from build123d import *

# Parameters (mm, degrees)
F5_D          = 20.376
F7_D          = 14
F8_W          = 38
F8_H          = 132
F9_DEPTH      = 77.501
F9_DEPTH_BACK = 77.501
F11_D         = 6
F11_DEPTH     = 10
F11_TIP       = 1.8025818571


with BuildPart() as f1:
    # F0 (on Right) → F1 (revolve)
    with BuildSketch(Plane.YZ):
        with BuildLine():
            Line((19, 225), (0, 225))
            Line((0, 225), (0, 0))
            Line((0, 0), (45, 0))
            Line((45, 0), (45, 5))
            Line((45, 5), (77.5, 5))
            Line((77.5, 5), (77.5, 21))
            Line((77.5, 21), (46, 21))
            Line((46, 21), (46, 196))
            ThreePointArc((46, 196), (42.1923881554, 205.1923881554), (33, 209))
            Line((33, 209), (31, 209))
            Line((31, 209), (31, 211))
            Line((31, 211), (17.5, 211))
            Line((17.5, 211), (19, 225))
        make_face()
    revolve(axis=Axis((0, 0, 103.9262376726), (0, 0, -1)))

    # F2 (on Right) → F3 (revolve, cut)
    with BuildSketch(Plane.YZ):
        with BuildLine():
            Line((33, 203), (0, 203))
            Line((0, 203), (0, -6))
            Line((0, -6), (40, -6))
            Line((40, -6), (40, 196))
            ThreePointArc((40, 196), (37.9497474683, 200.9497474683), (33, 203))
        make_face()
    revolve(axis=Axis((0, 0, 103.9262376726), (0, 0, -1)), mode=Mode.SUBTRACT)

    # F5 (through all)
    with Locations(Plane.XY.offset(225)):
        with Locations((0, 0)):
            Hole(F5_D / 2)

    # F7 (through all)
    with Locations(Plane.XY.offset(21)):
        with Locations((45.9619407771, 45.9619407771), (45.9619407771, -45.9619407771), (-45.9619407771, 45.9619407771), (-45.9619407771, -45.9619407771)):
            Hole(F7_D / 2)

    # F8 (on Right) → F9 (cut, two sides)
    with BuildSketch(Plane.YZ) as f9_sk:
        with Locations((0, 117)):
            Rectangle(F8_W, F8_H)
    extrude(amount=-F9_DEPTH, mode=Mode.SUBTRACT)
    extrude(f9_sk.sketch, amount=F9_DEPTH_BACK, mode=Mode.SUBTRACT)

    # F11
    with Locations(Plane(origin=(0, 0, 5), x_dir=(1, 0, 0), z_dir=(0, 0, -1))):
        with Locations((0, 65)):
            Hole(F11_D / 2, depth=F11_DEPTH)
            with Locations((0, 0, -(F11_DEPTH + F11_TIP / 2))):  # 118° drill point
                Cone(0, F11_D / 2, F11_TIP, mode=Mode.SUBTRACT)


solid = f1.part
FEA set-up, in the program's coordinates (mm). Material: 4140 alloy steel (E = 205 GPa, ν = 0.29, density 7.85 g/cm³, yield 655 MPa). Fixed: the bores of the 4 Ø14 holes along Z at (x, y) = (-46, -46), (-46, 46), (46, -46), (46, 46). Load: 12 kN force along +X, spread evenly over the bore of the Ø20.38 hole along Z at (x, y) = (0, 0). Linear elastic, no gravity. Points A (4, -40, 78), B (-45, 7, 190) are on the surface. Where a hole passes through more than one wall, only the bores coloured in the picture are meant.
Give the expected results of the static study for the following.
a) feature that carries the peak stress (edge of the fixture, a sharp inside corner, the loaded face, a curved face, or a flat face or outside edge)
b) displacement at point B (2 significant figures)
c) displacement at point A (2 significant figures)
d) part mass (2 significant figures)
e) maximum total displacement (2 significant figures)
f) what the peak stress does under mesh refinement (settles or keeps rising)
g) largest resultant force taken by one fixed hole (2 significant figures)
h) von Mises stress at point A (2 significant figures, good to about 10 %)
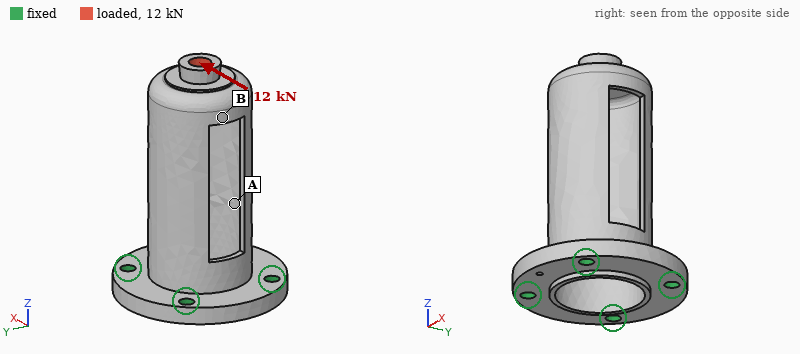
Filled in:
edge of the fixture
0.27 mm
0.059 mm
3.9 kg
0.34 mm
keeps rising
16 kN
34 MPa
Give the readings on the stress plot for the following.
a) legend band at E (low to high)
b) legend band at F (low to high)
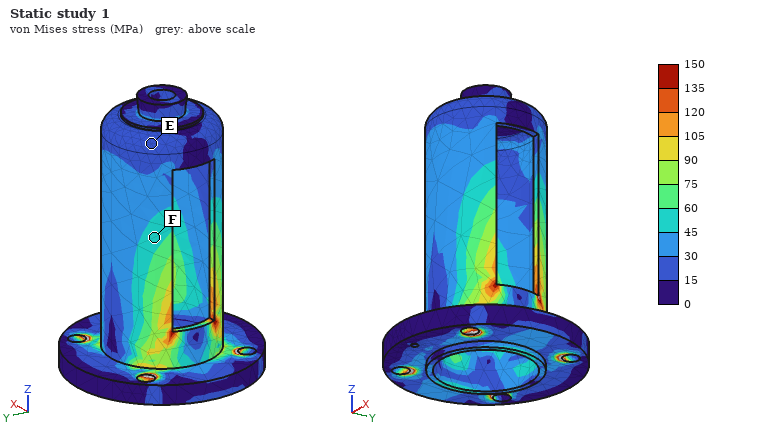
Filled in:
15 to 30 MPa
45 to 60 MPa
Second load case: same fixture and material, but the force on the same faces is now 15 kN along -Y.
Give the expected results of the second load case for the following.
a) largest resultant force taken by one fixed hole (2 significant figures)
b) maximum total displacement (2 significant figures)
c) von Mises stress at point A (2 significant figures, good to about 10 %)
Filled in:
19 kN
0.97 mm
89 MPa
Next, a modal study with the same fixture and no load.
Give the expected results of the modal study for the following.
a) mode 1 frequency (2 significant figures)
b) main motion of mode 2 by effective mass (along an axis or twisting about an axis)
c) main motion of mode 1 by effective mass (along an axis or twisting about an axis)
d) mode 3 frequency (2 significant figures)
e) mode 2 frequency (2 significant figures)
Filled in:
650 Hz
along X
along Y
1800 Hz
1100 Hz
